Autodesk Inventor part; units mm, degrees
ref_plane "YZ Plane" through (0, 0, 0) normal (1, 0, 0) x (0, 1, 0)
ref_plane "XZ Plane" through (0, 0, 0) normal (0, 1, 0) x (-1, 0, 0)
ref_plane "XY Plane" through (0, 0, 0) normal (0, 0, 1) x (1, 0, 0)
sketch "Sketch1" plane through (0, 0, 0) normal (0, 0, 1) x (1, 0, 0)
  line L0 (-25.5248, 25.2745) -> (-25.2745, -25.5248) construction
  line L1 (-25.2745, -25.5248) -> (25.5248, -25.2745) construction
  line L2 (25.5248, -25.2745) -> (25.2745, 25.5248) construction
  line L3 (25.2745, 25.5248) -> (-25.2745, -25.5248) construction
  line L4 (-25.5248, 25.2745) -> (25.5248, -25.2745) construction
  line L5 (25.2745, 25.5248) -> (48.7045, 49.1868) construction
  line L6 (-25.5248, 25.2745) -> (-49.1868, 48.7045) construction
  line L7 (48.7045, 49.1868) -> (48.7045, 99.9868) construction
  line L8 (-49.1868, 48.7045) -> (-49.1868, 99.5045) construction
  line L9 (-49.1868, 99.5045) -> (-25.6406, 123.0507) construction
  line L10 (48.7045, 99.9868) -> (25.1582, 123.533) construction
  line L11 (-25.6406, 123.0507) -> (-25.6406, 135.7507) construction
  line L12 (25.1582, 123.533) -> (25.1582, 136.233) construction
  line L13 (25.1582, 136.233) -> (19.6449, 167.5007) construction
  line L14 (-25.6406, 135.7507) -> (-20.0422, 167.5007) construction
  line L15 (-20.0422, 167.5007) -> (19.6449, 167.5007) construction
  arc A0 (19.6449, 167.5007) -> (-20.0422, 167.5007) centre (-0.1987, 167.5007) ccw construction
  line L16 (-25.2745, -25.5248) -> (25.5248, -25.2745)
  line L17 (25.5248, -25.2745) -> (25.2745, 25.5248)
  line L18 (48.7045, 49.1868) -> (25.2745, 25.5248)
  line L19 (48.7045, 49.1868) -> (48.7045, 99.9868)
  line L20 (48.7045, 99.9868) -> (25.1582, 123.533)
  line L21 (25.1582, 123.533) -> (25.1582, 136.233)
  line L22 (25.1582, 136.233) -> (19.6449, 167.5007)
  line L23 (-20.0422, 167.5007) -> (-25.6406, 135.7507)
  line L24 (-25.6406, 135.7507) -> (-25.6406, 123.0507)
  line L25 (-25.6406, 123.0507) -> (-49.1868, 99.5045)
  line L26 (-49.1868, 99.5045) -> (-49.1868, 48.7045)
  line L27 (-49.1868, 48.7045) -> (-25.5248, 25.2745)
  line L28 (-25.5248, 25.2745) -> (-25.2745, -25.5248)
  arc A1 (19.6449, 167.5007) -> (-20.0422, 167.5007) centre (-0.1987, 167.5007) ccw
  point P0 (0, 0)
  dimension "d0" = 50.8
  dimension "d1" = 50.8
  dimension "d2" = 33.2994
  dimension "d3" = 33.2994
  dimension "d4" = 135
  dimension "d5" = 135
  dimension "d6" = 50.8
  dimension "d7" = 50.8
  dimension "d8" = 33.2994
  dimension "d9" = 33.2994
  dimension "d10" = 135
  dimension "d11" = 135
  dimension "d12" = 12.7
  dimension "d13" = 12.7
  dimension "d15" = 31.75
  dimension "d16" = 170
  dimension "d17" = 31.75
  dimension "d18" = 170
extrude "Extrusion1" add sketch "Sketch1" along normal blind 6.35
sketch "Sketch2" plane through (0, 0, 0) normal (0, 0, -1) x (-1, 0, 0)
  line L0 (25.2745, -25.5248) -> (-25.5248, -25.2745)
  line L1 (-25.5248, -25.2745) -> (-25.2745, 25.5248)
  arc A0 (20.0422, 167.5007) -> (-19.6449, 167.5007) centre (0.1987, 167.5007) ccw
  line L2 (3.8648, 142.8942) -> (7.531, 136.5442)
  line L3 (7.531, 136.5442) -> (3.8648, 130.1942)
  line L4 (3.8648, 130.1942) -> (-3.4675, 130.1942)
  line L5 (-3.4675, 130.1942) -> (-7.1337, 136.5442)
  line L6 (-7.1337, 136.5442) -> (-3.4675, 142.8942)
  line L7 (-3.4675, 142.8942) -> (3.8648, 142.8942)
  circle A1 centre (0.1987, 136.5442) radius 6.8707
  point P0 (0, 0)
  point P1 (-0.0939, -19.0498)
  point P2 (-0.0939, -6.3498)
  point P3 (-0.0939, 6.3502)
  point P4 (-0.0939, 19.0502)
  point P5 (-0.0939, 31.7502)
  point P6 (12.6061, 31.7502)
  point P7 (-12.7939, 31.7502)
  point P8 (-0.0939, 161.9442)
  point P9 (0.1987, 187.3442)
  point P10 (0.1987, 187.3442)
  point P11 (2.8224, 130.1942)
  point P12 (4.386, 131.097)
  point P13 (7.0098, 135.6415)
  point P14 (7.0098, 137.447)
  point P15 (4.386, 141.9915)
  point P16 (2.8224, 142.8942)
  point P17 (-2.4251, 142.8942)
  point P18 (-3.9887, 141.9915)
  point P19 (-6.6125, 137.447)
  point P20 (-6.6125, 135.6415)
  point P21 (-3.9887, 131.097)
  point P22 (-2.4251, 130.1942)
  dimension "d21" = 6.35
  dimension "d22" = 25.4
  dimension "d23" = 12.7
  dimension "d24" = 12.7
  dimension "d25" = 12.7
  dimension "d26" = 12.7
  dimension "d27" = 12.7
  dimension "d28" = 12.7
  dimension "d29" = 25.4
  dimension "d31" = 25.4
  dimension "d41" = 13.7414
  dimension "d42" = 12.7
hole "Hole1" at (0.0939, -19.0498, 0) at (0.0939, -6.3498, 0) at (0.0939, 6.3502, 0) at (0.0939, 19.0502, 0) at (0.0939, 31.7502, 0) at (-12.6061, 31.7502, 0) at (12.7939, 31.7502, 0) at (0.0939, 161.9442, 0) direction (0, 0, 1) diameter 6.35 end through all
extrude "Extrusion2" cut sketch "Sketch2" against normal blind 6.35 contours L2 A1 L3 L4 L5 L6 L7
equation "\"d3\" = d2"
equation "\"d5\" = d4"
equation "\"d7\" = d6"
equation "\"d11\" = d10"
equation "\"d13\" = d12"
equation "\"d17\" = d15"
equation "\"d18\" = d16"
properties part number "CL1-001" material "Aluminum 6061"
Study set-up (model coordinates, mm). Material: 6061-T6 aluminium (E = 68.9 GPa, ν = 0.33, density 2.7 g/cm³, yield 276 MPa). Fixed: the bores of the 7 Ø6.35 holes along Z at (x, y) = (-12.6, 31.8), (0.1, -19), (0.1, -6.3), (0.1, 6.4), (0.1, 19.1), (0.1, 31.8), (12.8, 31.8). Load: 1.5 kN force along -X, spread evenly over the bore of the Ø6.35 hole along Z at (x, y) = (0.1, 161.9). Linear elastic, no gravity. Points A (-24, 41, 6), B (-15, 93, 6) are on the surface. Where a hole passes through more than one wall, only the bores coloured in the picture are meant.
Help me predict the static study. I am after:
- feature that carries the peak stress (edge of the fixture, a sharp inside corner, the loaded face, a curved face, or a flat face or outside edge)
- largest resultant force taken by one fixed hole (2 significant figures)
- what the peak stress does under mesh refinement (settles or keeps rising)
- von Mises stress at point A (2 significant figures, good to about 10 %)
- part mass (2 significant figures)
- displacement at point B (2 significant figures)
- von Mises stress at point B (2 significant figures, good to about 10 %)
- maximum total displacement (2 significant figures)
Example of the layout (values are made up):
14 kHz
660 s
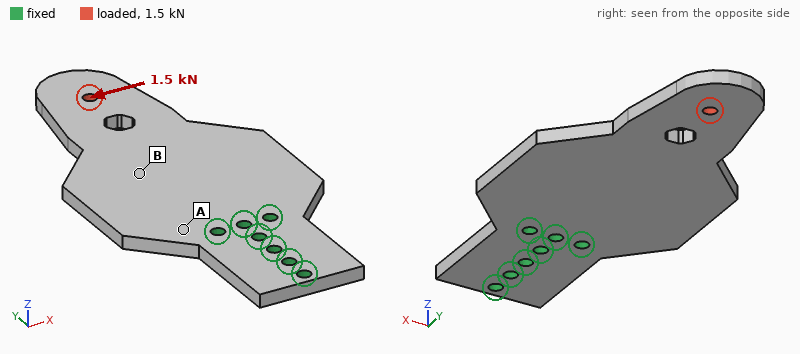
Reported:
edge of the fixture
4.4 kN
keeps rising
24 MPa
230 g
0.062 mm
8.1 MPa
0.19 mm
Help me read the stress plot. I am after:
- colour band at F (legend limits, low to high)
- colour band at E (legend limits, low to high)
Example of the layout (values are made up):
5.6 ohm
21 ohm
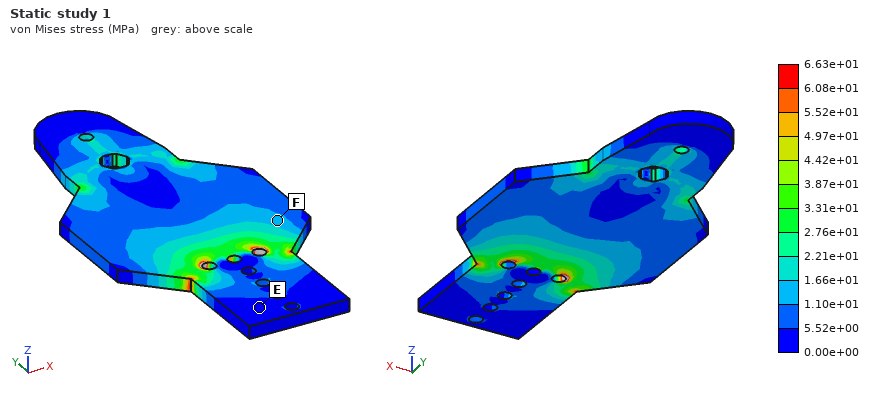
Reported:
1.10e+01 to 1.66e+01 MPa
0.00e+00 to 5.52e+00 MPa
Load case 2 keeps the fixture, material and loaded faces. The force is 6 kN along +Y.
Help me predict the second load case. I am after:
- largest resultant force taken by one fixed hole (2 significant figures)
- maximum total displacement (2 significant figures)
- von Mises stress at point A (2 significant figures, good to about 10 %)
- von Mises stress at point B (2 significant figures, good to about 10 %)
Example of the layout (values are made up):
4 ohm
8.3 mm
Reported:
2.1 kN
41 µm
11 MPa
14 MPa
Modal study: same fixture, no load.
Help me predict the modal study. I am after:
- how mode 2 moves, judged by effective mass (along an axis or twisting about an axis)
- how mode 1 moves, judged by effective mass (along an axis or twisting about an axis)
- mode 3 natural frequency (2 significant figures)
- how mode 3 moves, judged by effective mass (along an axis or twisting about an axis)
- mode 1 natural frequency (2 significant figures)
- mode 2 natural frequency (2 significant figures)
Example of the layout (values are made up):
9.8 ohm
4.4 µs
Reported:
twisting about Y
along Z
1300 Hz
along Z
310 Hz
1200 Hz
